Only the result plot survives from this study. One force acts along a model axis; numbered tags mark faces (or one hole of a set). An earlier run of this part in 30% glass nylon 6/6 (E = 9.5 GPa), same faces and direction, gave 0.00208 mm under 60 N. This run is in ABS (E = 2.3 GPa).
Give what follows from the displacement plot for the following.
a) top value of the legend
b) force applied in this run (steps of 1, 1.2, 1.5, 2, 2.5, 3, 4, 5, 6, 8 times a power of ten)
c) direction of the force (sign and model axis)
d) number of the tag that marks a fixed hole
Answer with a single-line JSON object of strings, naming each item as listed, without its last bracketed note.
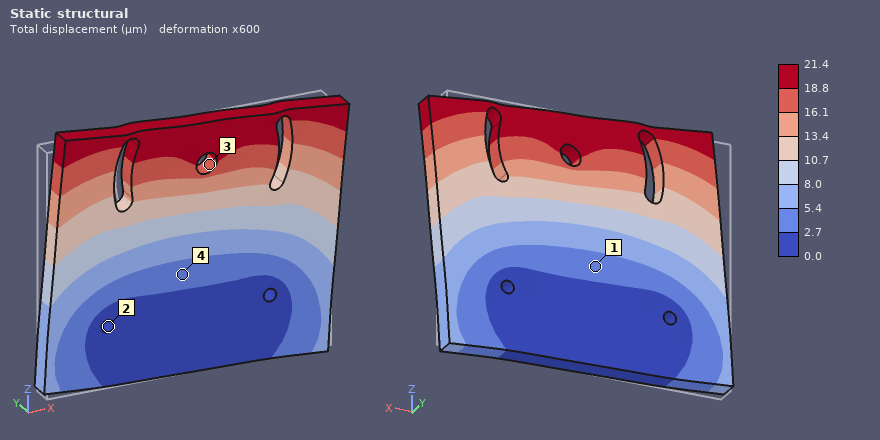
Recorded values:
{"top value of the legend": "21.4 µm", "force applied in this run": "150 N", "direction of the force": "+X", "number of the tag that marks a fixed hole": "2"}
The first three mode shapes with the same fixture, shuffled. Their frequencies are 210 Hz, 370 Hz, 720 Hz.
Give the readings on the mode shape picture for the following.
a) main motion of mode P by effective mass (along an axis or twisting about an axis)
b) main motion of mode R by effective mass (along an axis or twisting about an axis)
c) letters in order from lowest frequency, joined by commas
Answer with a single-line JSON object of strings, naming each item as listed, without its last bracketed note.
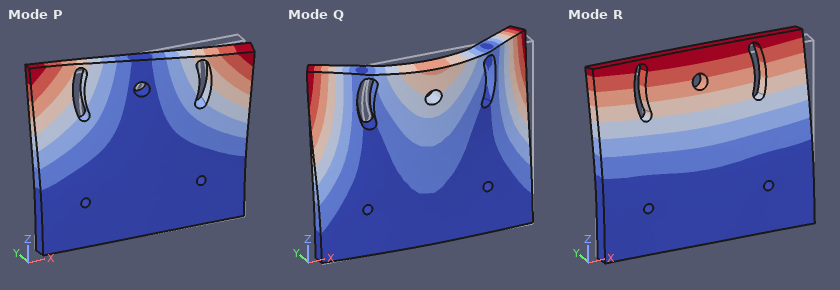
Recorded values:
{"main motion of mode P by effective mass": "twisting about Z", "main motion of mode R by effective mass": "along Y", "letters in order from lowest frequency, joined by commas": "R, P, Q"}
